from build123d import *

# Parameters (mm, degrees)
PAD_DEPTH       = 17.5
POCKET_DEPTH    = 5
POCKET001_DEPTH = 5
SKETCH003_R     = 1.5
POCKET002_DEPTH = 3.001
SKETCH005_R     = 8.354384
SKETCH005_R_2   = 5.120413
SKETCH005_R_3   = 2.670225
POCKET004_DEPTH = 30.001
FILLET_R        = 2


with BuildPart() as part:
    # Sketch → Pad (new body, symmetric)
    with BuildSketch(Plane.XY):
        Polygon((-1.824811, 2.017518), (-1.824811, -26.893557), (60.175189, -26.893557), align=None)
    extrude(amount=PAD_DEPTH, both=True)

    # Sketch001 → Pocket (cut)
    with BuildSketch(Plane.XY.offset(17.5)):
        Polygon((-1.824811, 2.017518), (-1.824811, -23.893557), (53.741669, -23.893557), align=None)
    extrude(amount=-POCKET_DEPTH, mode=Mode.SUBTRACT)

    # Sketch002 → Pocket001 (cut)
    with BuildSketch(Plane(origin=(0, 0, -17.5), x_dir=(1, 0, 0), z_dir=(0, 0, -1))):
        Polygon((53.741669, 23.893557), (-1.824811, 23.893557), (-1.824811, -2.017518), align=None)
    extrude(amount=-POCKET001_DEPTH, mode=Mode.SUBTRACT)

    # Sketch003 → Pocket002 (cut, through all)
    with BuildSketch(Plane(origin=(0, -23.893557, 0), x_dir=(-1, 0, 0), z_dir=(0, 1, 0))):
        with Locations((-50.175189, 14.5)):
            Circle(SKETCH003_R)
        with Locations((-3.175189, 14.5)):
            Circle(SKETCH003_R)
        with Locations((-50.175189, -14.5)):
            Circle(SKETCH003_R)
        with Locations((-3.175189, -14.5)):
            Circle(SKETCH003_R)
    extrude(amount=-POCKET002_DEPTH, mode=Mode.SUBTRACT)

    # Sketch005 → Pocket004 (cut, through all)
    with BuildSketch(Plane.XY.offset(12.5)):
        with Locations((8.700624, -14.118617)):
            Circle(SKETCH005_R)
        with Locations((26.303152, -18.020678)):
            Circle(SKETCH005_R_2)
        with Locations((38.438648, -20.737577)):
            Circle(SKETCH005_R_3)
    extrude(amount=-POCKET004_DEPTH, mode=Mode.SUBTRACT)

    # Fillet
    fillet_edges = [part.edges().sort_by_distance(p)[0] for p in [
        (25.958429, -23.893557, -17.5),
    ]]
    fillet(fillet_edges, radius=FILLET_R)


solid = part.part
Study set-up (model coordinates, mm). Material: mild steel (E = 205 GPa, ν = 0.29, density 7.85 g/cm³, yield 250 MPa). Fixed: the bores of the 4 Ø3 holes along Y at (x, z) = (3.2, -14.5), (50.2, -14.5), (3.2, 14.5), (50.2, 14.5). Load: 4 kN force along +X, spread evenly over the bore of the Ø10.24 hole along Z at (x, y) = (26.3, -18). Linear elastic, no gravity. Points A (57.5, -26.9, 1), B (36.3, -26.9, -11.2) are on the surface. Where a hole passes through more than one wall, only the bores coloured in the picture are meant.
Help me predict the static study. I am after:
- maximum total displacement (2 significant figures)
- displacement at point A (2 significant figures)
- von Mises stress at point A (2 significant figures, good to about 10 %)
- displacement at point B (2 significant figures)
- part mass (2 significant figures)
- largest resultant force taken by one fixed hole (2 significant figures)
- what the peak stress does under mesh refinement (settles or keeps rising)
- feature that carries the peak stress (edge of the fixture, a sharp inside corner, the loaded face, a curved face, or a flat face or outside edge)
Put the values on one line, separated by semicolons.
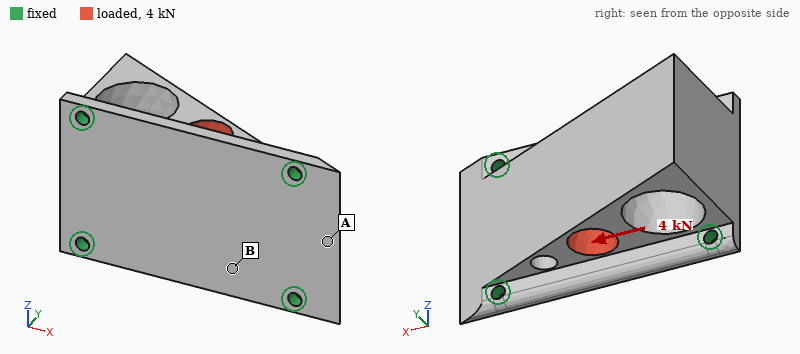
5.4 µm; 2.3 µm; 20 MPa; 1.6 µm; 130 g; 1.1 kN; keeps rising; edge of the fixture
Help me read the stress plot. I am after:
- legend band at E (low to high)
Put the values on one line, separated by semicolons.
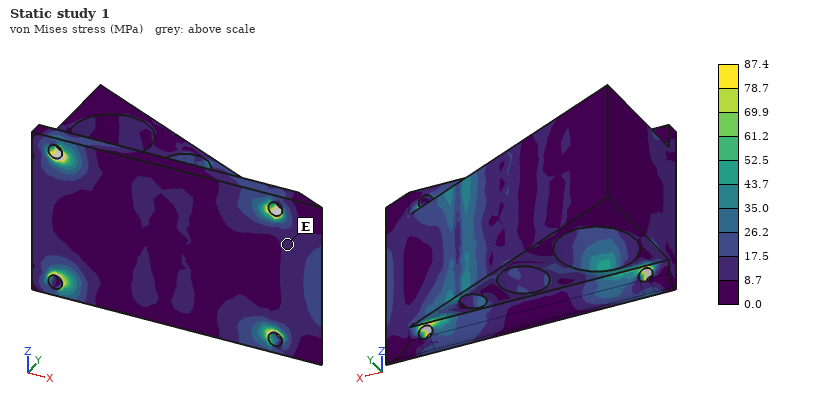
8.7 to 17.5 MPa
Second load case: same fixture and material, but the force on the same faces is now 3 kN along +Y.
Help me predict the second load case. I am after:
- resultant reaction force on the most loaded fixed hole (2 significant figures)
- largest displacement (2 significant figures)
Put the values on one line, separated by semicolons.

1.0 kN; 16 µm
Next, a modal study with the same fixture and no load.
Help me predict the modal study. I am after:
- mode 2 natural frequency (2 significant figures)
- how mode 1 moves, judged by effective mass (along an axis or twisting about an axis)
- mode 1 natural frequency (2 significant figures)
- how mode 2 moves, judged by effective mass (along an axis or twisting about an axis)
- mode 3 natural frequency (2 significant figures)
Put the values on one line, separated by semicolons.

10 kHz; along Y; 9000 Hz; along Z; 12 kHz
